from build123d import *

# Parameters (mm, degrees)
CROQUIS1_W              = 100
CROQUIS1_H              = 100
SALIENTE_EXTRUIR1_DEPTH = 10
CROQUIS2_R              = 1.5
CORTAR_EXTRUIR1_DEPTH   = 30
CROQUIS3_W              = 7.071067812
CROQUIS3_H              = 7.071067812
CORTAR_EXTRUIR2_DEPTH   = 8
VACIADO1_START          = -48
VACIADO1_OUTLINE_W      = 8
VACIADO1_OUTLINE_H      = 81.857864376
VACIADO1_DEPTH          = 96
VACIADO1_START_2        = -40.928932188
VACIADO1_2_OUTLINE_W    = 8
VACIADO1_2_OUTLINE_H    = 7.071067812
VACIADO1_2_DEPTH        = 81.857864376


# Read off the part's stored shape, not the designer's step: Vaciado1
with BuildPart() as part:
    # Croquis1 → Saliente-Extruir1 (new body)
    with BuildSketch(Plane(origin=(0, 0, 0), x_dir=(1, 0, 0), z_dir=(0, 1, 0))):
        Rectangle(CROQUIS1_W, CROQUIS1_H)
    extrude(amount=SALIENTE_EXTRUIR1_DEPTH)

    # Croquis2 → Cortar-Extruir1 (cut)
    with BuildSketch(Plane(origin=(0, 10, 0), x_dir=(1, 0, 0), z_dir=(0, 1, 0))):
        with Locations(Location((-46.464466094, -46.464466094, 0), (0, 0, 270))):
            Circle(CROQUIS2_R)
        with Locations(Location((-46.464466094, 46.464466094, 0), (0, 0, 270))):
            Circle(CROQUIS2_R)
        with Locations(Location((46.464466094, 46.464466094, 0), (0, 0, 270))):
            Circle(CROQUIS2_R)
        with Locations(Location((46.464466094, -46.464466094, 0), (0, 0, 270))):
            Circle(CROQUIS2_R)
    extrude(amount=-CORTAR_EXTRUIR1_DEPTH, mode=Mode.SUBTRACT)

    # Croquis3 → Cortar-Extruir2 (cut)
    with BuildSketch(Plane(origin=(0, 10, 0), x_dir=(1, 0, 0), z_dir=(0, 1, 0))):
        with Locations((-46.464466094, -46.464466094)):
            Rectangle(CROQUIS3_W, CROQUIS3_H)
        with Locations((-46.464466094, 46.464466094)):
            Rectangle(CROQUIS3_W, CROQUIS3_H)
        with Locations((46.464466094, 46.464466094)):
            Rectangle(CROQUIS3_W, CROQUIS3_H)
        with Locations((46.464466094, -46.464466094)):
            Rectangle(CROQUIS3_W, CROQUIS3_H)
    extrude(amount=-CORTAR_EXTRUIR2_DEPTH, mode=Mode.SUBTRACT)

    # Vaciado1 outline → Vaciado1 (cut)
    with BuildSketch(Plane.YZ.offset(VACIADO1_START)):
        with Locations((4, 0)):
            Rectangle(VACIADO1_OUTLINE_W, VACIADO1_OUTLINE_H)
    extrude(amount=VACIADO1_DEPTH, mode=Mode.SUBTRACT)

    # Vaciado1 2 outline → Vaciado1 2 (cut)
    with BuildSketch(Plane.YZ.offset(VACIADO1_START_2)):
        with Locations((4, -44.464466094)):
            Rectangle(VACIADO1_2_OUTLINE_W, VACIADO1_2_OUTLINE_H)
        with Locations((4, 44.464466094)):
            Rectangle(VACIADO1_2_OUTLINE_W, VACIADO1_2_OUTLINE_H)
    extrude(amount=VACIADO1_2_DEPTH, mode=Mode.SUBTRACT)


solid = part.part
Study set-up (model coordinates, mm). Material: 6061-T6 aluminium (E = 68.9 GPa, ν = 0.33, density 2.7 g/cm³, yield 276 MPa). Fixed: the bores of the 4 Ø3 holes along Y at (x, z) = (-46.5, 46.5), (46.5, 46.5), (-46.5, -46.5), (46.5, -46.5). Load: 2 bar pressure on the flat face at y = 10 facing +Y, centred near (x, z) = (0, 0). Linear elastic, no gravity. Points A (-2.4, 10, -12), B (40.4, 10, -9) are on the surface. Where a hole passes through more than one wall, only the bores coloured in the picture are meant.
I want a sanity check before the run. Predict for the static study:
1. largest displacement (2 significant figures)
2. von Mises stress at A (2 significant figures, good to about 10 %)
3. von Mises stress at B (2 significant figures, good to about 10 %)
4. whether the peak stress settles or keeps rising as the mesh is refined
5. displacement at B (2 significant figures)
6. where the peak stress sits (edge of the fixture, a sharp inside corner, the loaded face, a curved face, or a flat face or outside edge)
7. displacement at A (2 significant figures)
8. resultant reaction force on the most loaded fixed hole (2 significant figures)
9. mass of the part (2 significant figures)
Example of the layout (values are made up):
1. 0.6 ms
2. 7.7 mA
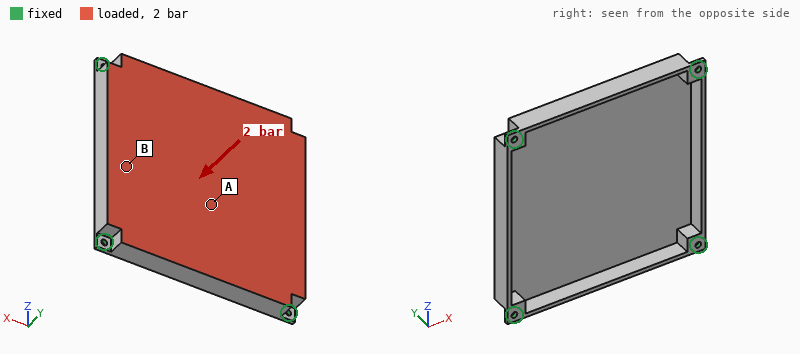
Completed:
1. 1.0 mm
2. 110 MPa
3. 45 MPa
4. keeps rising
5. 0.30 mm
6. edge of the fixture
7. 0.97 mm
8. 1.0 kN
9. 71 g
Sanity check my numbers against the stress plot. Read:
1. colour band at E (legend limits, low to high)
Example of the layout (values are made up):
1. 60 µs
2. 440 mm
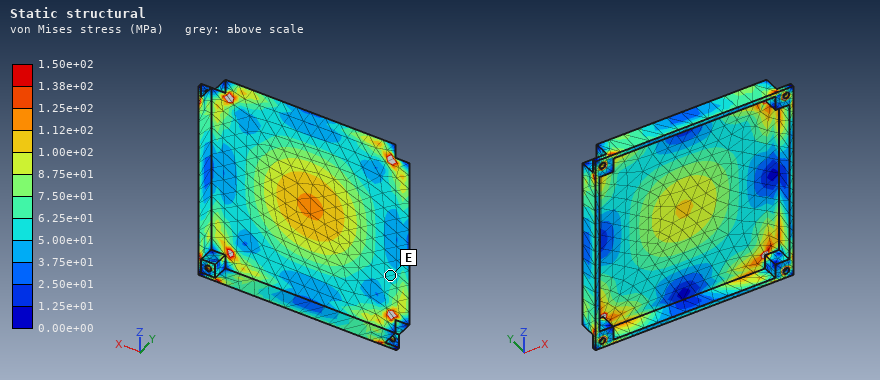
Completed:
1. 5.00e+01 to 6.25e+01 MPa
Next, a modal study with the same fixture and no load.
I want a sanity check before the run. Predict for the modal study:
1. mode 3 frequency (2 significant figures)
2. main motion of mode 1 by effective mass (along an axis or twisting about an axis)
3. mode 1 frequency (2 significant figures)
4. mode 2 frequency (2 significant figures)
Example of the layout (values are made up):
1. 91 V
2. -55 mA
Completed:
1. 2600 Hz
2. along Y
3. 1200 Hz
4. 2600 Hz
